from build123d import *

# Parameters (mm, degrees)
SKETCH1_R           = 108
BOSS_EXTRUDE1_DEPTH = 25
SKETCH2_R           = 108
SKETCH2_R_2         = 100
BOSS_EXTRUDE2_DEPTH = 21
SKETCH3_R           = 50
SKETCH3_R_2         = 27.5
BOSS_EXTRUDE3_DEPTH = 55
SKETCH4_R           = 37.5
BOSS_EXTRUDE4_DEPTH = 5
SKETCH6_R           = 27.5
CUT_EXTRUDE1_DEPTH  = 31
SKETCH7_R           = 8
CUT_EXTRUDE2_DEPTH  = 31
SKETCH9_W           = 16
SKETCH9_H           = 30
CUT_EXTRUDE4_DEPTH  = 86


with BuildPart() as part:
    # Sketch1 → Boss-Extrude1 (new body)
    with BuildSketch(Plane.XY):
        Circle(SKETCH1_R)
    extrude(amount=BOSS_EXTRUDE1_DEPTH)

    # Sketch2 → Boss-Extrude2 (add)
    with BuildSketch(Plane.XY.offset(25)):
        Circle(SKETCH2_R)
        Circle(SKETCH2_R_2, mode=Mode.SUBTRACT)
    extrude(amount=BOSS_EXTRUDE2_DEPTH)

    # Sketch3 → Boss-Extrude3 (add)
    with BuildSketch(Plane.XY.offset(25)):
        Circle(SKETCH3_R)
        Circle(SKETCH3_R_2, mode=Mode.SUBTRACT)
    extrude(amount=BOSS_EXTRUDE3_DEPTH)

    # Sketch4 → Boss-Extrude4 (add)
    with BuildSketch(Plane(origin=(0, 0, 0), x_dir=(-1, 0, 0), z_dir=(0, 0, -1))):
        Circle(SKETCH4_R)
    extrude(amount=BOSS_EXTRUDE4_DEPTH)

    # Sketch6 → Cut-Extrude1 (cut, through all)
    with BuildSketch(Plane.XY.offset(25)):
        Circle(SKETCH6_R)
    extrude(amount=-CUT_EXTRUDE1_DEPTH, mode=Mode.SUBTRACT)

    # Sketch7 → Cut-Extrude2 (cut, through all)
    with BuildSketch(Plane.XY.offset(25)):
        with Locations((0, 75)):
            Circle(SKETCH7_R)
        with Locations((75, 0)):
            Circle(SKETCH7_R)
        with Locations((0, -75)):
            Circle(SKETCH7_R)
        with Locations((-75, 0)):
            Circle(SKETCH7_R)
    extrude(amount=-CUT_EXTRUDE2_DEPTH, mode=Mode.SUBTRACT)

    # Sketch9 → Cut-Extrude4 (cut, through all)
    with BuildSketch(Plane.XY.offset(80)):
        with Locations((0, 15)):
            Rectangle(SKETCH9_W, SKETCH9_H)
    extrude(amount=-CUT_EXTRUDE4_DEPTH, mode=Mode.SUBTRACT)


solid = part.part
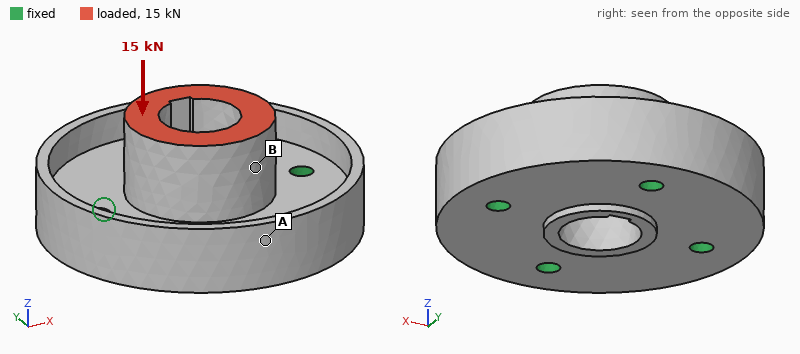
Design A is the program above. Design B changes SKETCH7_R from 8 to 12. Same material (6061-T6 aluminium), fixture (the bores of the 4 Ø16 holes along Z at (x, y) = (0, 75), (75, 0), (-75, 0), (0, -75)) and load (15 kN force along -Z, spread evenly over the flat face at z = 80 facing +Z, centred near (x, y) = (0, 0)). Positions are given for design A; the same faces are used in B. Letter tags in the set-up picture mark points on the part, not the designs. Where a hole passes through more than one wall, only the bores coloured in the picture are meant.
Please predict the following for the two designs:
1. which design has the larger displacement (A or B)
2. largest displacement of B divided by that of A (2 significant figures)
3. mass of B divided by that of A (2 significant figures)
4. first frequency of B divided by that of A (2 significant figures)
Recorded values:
A
0.81
0.98
1.2
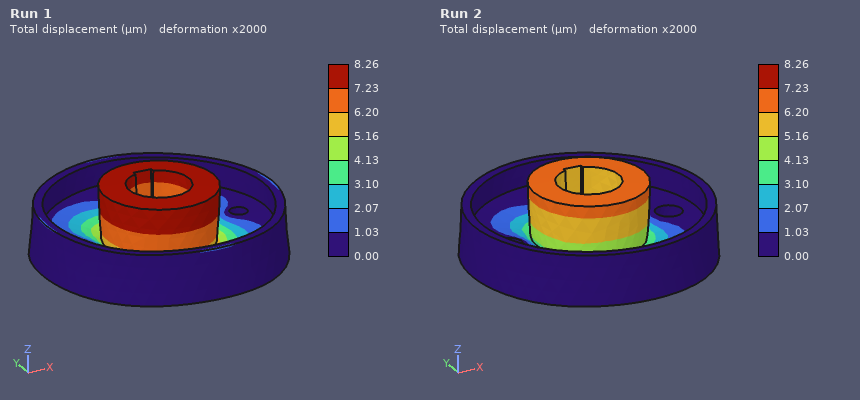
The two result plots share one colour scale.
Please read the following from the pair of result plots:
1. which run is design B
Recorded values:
Run 2
